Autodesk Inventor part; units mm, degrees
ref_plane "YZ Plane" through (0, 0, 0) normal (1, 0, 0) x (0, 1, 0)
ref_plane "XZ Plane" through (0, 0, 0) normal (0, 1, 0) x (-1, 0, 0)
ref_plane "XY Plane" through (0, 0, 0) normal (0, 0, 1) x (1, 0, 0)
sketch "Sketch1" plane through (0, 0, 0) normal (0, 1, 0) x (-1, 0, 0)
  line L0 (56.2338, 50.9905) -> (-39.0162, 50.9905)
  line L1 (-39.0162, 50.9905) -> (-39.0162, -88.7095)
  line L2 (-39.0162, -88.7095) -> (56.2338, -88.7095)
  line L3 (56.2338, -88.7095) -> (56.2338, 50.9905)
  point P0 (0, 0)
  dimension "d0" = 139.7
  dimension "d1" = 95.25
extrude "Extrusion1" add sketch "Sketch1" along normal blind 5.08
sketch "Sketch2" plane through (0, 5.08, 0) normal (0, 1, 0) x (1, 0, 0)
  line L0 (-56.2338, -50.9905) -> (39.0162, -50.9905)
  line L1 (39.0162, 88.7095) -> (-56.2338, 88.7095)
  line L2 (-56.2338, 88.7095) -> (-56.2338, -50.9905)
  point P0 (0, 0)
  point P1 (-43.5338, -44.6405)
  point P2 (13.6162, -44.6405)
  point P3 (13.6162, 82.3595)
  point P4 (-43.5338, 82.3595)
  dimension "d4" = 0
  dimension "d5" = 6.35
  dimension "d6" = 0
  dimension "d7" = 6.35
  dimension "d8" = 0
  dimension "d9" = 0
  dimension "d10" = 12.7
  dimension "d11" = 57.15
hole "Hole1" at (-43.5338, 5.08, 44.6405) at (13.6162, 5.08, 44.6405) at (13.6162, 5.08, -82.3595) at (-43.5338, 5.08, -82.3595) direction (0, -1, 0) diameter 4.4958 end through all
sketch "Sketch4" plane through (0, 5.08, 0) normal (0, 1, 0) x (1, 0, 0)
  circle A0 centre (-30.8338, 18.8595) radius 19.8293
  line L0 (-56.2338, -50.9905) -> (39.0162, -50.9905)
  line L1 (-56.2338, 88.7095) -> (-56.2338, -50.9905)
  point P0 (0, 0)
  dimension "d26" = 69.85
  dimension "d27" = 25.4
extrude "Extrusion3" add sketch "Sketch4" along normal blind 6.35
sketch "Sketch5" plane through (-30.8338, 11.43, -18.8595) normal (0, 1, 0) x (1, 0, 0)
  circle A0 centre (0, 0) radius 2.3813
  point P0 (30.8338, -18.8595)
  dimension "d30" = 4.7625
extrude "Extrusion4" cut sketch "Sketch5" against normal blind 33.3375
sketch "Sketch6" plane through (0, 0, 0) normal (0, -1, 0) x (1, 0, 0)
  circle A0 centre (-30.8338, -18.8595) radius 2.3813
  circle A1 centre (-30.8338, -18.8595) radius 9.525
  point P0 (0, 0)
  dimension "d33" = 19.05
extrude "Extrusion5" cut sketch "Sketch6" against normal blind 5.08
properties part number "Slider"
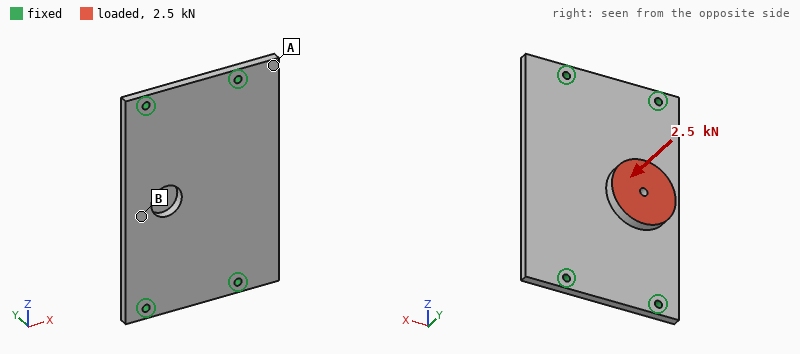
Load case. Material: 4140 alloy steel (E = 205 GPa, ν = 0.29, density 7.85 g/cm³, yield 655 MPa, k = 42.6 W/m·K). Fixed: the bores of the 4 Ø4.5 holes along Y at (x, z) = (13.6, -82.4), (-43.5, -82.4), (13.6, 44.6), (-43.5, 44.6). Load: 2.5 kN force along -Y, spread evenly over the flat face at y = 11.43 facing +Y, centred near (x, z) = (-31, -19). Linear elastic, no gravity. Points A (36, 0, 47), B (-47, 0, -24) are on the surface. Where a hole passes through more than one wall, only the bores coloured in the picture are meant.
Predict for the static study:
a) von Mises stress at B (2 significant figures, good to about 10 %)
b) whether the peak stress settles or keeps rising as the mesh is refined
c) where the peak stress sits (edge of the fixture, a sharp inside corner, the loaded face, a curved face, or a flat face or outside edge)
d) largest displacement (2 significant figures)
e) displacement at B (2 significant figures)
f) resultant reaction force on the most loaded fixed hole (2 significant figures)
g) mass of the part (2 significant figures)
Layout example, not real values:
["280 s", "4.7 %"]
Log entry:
["48 MPa", "keeps rising", "edge of the fixture", "0.16 mm", "0.14 mm", "1.3 kN", "580 g"]
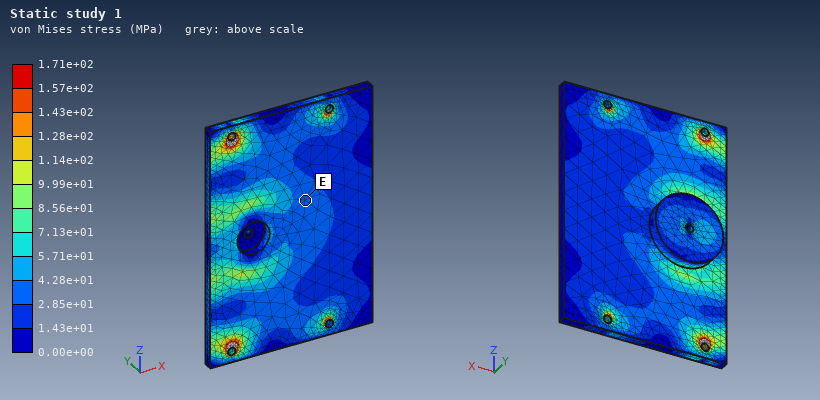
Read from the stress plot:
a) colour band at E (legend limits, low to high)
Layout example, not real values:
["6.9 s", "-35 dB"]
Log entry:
["2.85e+01 to 4.28e+01 MPa"]
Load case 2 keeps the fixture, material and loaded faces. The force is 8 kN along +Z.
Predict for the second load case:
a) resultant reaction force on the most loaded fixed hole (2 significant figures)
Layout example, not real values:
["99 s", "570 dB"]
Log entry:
["2.4 kN"]
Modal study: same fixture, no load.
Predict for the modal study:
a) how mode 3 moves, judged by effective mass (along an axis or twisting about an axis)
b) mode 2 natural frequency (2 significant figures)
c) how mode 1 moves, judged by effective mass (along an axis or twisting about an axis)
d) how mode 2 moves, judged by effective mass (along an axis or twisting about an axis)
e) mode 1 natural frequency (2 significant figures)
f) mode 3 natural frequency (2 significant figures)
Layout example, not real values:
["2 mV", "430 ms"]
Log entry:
["twisting about X", "1900 Hz", "along Y", "twisting about Z", "1400 Hz", "3800 Hz"]
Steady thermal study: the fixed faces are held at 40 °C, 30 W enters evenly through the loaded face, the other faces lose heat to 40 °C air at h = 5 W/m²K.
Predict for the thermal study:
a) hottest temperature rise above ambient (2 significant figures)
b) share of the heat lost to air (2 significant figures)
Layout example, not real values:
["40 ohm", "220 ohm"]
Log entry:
["61 K", "12 %"]
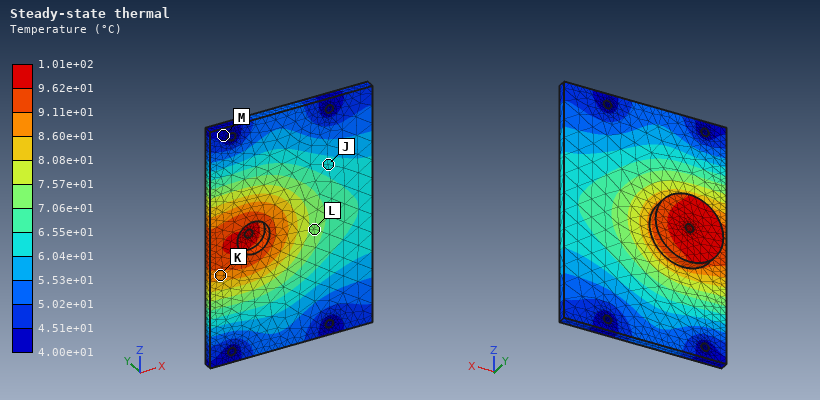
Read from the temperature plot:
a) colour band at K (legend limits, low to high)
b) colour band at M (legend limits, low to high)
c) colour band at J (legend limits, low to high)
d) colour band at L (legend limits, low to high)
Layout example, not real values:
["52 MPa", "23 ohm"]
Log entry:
["8.60e+01 to 9.11e+01 °C", "4.00e+01 to 4.51e+01 °C", "6.04e+01 to 6.55e+01 °C", "7.06e+01 to 7.57e+01 °C"]
